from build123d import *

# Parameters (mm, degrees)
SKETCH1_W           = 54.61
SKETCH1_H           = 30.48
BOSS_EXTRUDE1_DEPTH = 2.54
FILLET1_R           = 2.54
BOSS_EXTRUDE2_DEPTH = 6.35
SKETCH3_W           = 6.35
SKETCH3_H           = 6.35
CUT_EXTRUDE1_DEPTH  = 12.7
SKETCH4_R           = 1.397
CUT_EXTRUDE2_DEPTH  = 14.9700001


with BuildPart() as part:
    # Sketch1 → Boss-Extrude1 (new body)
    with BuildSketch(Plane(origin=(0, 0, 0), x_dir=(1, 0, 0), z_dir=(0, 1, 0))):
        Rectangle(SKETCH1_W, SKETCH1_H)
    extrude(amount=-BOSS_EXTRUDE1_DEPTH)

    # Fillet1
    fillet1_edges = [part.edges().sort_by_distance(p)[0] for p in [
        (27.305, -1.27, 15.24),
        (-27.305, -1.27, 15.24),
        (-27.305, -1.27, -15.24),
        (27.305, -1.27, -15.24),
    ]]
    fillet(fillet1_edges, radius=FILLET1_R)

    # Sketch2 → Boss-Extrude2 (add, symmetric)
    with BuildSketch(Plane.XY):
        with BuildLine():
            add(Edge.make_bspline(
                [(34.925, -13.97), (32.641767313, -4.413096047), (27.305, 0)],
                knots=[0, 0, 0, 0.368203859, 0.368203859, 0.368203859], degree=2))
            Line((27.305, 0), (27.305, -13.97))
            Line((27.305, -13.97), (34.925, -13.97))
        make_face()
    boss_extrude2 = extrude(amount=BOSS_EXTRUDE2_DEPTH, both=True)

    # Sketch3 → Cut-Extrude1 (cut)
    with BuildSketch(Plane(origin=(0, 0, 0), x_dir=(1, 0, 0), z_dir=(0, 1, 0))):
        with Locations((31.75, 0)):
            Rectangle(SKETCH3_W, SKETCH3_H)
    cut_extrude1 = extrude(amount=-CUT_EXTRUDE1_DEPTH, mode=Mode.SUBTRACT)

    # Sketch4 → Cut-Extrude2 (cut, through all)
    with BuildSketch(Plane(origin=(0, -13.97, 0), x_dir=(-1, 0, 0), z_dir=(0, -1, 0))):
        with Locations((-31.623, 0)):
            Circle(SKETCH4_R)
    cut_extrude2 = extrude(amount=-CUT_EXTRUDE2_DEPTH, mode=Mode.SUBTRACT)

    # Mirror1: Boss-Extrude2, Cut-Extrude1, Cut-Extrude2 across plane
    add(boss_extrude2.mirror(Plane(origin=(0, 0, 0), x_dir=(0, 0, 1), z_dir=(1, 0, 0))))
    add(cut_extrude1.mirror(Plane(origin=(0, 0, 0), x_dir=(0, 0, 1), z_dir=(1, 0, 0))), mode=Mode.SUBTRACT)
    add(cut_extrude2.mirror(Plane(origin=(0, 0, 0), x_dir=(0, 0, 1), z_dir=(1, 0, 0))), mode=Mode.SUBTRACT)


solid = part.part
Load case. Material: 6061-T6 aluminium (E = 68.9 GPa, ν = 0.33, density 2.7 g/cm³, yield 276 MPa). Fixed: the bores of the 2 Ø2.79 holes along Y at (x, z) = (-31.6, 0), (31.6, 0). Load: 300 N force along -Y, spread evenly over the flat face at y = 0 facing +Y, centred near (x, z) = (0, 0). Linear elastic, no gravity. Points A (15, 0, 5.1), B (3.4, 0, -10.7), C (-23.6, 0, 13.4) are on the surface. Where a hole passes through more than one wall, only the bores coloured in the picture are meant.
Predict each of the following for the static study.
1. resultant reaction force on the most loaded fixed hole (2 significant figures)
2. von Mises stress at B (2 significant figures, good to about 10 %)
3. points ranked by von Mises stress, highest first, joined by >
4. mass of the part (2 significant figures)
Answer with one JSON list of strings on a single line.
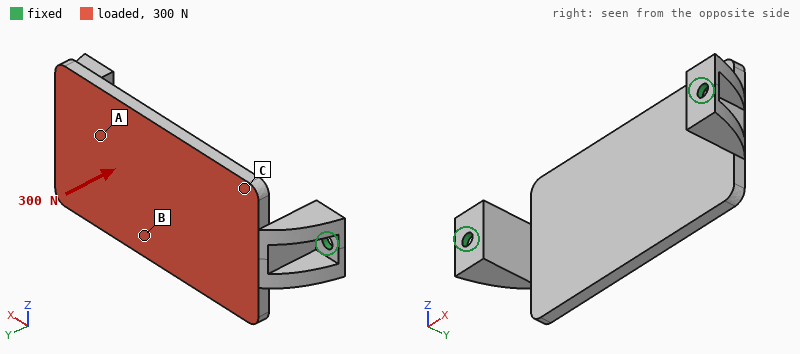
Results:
["190 N", "37 MPa", "B > A > C", "14 g"]
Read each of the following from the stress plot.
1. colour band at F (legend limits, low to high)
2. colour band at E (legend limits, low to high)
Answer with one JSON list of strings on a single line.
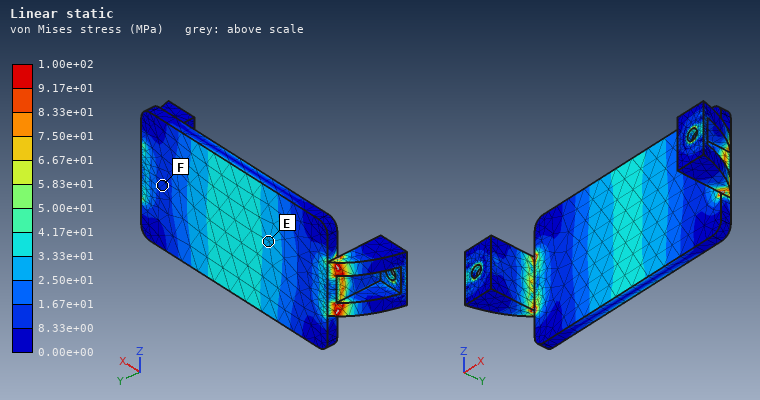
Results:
["8.33e+00 to 1.67e+01 MPa", "2.50e+01 to 3.33e+01 MPa"]
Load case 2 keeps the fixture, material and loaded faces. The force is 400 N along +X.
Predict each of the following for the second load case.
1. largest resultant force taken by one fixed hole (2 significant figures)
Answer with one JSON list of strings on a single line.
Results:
["200 N"]
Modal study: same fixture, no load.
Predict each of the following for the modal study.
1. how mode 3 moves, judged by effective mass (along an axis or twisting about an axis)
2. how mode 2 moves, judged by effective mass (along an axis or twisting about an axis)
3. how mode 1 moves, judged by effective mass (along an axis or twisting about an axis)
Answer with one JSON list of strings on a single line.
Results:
["along X", "along Y", "along Z"]
